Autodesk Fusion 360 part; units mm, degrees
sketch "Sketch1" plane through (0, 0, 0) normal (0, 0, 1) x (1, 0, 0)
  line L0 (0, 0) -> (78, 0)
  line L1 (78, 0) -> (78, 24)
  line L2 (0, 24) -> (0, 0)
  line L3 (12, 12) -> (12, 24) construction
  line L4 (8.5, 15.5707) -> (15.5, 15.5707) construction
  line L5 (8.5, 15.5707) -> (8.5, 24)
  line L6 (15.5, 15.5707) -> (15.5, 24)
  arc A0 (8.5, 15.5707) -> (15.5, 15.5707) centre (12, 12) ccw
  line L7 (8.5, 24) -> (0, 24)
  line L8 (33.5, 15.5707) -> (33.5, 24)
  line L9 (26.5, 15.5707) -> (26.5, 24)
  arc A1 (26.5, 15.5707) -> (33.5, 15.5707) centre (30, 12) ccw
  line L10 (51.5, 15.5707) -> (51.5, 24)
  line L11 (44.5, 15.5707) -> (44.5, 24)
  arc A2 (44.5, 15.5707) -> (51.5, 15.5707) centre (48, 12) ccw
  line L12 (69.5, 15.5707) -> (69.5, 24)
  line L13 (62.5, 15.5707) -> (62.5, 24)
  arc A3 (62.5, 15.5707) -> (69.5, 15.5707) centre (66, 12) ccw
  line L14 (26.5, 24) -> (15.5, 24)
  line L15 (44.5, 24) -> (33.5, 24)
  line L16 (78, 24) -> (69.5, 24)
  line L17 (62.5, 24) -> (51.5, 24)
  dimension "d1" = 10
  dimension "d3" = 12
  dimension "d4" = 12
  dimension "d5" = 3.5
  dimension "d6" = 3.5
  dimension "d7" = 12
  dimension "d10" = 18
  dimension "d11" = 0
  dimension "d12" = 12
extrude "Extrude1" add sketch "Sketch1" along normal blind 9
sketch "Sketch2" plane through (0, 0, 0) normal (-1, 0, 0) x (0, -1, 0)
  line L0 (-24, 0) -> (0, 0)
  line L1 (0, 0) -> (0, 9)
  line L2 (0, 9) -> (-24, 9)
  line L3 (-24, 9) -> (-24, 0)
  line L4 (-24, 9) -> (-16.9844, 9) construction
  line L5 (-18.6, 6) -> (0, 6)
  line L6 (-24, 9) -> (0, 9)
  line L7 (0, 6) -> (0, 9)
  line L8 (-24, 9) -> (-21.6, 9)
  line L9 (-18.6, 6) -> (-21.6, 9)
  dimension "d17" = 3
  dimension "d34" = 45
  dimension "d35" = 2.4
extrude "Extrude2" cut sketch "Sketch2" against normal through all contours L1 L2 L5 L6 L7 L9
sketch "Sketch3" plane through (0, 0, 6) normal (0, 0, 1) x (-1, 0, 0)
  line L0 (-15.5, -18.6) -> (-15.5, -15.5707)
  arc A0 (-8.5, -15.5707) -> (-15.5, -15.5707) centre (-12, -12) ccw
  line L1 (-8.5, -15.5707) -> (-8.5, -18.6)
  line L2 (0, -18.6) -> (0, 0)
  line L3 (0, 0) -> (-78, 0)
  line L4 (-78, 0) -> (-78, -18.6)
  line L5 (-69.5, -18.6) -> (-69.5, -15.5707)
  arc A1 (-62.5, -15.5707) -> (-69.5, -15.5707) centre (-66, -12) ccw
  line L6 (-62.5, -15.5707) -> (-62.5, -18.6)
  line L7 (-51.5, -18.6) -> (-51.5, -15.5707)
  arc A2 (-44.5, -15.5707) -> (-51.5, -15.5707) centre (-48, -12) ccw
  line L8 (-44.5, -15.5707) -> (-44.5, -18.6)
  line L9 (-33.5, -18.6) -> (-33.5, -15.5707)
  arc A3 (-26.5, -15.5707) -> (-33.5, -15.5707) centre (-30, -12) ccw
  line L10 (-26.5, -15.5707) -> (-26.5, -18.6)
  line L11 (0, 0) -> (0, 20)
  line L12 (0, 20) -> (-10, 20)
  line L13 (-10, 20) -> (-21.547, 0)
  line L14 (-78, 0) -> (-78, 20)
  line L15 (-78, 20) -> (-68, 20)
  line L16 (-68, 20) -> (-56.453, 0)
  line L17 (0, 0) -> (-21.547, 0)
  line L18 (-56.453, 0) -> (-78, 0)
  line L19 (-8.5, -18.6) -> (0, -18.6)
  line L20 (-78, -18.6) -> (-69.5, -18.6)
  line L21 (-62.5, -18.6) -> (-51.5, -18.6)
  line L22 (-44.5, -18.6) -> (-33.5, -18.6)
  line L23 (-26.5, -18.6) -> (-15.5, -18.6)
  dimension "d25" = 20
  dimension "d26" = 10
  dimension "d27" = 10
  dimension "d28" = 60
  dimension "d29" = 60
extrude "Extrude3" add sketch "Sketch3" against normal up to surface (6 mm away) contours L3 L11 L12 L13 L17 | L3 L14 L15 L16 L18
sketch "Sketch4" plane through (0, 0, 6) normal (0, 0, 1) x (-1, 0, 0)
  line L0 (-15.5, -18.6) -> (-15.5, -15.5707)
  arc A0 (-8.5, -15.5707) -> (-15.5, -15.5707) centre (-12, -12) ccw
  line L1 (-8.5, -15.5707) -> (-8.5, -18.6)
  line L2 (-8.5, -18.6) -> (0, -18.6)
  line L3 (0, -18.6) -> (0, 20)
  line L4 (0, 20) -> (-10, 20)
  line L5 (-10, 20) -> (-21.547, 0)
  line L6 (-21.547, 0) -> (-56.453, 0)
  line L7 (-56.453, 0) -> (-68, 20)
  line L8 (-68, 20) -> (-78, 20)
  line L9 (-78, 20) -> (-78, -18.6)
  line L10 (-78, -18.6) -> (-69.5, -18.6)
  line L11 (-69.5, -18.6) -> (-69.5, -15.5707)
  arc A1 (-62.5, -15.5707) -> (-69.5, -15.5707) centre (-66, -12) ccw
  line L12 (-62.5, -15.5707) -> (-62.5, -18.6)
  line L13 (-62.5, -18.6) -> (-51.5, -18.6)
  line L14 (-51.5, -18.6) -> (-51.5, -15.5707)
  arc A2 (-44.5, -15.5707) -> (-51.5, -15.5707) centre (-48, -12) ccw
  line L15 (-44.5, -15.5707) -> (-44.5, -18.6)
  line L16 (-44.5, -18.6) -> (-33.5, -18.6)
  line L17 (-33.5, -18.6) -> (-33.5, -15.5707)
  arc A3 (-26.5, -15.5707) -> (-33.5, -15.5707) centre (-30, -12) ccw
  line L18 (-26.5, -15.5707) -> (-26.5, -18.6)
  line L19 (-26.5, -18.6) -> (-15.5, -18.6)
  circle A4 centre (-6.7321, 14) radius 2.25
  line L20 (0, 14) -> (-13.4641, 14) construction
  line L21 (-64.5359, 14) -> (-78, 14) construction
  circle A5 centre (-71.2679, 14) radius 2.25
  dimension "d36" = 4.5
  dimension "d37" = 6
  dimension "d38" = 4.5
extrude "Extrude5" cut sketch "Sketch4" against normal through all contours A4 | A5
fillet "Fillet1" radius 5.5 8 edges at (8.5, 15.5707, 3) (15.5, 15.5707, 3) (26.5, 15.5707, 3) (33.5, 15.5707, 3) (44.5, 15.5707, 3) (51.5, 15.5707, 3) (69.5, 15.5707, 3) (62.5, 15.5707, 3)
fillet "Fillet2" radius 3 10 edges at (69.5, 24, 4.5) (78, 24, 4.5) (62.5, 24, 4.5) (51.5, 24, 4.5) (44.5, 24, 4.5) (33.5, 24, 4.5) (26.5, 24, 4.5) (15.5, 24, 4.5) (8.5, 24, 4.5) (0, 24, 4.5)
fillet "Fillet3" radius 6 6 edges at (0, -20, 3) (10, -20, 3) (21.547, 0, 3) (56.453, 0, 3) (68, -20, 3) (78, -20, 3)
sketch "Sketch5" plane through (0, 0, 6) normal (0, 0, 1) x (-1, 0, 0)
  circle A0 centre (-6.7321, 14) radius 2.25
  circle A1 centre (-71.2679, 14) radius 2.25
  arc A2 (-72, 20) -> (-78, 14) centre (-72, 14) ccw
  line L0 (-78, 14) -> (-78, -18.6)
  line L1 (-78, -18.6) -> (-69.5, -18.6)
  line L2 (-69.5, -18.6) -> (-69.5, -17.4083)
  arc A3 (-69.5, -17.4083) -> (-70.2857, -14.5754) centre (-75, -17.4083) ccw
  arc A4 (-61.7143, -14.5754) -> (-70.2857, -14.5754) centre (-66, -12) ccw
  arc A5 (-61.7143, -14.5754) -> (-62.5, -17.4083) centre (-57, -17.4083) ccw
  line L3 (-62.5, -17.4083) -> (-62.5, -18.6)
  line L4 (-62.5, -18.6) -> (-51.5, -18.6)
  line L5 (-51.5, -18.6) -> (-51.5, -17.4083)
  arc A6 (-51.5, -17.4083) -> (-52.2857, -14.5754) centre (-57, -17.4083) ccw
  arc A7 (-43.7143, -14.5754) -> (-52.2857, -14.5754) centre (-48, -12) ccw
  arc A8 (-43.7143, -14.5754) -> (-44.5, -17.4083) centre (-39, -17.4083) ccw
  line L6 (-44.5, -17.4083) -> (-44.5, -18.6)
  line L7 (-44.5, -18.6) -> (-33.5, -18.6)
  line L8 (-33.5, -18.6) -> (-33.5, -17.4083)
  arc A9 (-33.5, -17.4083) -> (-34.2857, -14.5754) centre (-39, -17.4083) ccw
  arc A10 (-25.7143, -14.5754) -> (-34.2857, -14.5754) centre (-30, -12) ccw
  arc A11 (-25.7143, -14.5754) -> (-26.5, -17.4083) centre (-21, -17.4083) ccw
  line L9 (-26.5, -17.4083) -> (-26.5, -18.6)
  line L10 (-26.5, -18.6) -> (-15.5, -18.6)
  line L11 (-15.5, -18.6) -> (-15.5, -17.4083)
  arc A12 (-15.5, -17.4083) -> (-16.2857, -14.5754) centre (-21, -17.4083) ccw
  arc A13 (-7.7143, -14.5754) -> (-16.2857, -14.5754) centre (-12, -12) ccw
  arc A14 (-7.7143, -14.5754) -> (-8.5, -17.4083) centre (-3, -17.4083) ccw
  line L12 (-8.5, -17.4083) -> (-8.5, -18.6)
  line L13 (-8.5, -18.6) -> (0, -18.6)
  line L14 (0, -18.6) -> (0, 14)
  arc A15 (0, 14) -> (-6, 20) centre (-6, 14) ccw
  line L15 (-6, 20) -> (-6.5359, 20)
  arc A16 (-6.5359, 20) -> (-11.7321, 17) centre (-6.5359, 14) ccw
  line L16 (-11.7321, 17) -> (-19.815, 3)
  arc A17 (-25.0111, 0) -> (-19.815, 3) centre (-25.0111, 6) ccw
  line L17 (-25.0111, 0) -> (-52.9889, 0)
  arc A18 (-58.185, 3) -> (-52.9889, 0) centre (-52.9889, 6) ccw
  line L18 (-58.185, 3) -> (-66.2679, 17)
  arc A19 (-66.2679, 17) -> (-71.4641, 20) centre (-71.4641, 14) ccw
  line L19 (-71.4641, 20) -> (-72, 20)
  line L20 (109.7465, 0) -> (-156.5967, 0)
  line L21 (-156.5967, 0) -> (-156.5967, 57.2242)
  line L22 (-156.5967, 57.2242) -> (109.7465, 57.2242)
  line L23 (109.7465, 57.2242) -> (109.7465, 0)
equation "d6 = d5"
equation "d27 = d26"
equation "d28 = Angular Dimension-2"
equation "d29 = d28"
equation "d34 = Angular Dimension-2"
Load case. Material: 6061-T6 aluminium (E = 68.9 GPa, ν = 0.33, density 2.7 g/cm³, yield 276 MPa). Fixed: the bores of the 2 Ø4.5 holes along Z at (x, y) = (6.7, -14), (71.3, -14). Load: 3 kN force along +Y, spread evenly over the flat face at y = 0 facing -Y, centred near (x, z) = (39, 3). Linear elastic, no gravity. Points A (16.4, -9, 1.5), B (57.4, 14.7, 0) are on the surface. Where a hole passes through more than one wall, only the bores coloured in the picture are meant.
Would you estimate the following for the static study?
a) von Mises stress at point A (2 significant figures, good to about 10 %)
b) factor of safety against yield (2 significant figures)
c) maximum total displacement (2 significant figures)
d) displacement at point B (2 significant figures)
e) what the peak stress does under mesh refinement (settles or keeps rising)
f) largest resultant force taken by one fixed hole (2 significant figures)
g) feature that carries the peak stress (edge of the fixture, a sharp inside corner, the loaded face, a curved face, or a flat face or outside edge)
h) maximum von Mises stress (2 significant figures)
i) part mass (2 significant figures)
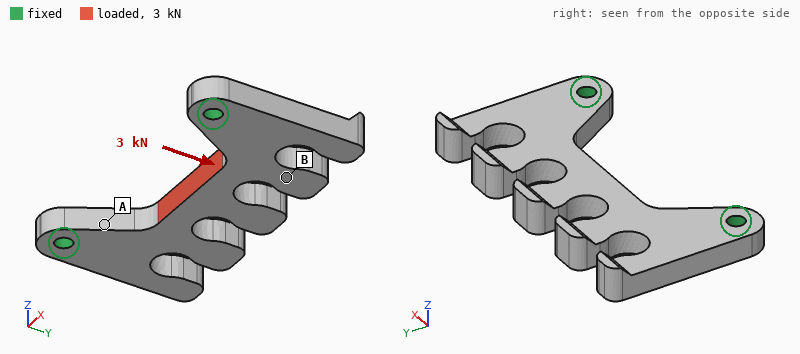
64 MPa
1.4
80 µm
48 µm
settles
2.1 kN
a curved face
200 MPa
32 g
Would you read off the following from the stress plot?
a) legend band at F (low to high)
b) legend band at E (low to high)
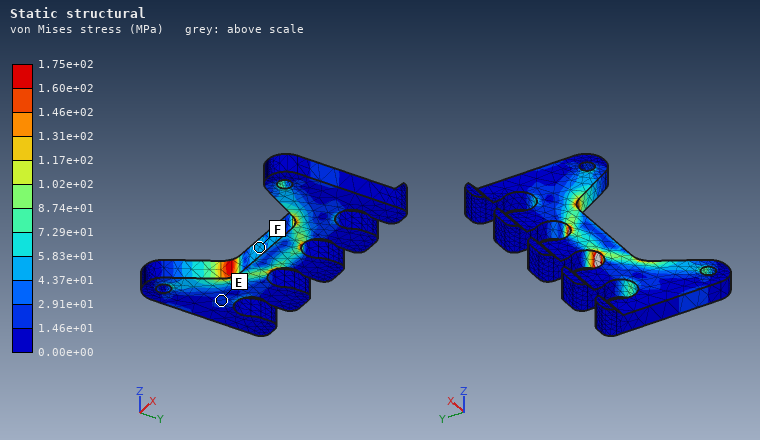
4.37e+01 to 5.83e+01 MPa
1.46e+01 to 2.91e+01 MPa
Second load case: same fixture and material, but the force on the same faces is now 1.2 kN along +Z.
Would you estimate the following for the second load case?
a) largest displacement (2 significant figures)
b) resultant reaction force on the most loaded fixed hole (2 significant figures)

0.22 mm
600 N
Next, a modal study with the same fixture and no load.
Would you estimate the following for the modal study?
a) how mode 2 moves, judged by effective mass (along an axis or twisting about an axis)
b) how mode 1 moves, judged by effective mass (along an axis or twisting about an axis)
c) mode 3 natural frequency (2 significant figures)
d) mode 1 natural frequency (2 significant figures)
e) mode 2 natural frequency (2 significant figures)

twisting about Y
along Z
5000 Hz
2300 Hz
3700 Hz
